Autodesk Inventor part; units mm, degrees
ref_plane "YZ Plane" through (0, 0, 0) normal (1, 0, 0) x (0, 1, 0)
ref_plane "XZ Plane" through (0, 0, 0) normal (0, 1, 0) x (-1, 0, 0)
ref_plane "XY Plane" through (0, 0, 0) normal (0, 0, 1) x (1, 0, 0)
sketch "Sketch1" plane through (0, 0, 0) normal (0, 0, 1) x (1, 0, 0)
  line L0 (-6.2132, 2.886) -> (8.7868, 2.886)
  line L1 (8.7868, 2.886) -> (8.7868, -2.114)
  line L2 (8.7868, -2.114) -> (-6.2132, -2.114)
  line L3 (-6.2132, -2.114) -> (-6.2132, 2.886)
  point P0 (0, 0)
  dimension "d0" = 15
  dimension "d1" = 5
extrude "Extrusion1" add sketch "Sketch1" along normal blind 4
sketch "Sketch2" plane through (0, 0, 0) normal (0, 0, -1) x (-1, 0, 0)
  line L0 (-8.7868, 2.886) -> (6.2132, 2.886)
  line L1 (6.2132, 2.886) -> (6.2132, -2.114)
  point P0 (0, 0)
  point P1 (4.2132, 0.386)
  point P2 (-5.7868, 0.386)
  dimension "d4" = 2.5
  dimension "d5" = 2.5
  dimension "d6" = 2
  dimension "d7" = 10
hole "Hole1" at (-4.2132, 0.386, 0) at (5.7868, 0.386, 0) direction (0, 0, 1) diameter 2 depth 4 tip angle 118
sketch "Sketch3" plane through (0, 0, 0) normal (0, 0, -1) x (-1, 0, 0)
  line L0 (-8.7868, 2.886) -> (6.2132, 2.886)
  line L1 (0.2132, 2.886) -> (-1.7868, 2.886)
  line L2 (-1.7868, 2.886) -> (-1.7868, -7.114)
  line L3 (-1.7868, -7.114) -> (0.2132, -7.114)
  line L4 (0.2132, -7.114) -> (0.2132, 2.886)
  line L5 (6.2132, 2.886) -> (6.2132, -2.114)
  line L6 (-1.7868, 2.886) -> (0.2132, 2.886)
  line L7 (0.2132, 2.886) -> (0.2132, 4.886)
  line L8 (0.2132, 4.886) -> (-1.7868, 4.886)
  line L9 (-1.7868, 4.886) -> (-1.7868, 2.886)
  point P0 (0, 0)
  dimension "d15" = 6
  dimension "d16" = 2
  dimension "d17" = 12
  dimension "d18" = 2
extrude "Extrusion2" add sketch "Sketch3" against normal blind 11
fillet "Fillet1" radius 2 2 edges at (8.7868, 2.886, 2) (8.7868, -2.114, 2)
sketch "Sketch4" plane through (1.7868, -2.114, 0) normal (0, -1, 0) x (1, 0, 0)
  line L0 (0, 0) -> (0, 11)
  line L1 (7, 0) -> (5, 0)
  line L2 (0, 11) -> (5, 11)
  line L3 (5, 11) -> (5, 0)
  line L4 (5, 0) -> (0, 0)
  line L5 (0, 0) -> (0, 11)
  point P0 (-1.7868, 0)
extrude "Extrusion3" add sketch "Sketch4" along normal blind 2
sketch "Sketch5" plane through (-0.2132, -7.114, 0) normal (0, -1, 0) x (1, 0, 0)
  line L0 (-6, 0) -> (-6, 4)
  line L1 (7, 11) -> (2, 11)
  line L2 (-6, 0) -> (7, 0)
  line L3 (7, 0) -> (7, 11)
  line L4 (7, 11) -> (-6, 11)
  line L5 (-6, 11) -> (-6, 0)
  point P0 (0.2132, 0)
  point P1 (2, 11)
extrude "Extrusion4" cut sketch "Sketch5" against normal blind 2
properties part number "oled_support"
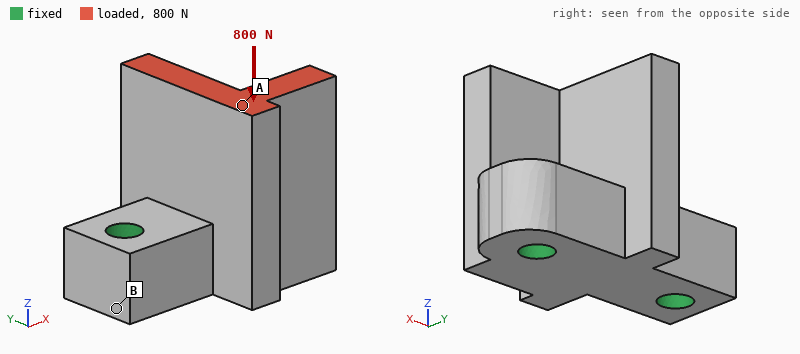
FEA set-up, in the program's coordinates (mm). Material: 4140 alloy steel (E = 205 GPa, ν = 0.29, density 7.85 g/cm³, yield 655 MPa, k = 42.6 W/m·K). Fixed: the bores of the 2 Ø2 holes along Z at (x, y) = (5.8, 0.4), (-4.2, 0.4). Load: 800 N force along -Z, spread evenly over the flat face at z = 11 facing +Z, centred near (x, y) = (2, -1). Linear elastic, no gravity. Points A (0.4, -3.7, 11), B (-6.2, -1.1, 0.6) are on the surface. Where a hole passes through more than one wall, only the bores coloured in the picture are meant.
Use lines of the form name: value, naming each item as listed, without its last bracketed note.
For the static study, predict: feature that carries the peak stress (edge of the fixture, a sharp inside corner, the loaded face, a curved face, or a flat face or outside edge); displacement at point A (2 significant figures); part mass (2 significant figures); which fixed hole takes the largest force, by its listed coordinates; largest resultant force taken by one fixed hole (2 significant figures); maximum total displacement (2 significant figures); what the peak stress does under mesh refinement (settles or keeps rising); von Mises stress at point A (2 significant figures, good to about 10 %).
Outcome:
feature that carries the peak stress: edge of the fixture
displacement at point A: 4.3 µm
part mass: 4.4 g
which fixed hole takes the largest force, by its listed coordinates: (5.8, 0.4)
largest resultant force taken by one fixed hole: 510 N
maximum total displacement: 4.7 µm
what the peak stress does under mesh refinement: keeps rising
von Mises stress at point A: 27 MPa
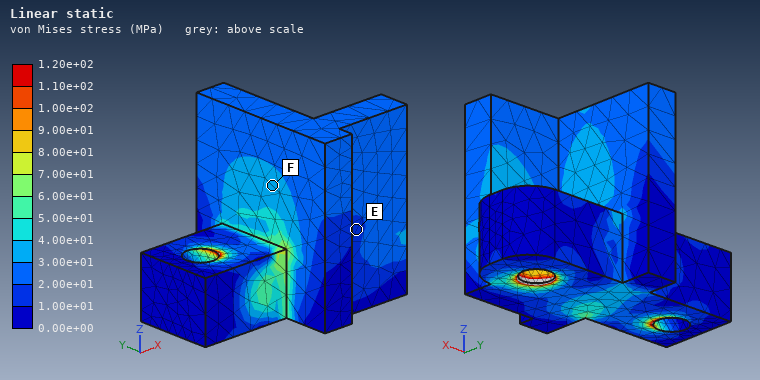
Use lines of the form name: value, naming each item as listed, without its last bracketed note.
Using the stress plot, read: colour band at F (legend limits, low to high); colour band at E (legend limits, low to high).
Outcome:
colour band at F: 3.00e+01 to 4.00e+01 MPa
colour band at E: 1.00e+01 to 2.00e+01 MPa
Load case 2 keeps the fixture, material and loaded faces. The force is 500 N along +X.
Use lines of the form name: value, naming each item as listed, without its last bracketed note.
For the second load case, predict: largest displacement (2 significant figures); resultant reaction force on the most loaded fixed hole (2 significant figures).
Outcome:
largest displacement: 27 µm
resultant reaction force on the most loaded fixed hole: 530 N
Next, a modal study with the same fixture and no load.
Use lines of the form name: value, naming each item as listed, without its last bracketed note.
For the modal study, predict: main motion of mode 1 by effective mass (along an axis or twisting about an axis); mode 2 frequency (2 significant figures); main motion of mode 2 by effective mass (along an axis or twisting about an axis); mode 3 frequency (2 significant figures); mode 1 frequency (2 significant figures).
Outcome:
main motion of mode 1 by effective mass: along Y
mode 2 frequency: 35 kHz
main motion of mode 2 by effective mass: along X
mode 3 frequency: 48 kHz
mode 1 frequency: 27 kHz
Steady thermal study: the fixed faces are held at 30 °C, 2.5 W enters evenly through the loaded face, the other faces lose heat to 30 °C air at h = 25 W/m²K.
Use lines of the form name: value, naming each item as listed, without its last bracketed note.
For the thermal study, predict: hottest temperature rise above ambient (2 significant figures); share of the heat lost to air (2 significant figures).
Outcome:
hottest temperature rise above ambient: 20 K
share of the heat lost to air: 3.8 %
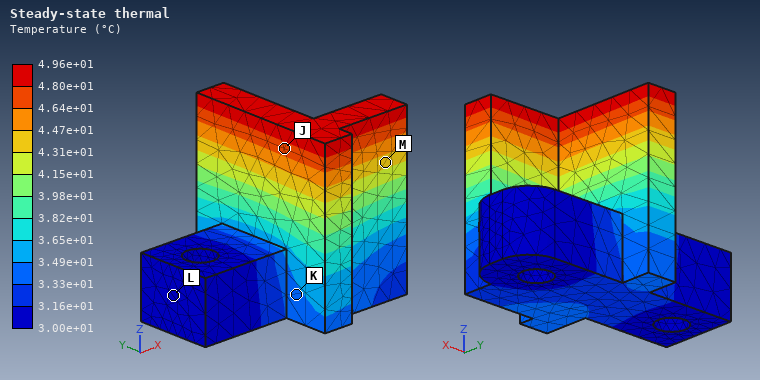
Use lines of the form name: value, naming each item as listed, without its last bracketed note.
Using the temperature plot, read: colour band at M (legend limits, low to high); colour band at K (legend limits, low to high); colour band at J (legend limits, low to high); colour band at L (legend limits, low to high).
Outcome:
colour band at M: 4.31e+01 to 4.47e+01 °C
colour band at K: 3.33e+01 to 3.49e+01 °C
colour band at J: 4.64e+01 to 4.80e+01 °C
colour band at L: 3.00e+01 to 3.16e+01 °C
